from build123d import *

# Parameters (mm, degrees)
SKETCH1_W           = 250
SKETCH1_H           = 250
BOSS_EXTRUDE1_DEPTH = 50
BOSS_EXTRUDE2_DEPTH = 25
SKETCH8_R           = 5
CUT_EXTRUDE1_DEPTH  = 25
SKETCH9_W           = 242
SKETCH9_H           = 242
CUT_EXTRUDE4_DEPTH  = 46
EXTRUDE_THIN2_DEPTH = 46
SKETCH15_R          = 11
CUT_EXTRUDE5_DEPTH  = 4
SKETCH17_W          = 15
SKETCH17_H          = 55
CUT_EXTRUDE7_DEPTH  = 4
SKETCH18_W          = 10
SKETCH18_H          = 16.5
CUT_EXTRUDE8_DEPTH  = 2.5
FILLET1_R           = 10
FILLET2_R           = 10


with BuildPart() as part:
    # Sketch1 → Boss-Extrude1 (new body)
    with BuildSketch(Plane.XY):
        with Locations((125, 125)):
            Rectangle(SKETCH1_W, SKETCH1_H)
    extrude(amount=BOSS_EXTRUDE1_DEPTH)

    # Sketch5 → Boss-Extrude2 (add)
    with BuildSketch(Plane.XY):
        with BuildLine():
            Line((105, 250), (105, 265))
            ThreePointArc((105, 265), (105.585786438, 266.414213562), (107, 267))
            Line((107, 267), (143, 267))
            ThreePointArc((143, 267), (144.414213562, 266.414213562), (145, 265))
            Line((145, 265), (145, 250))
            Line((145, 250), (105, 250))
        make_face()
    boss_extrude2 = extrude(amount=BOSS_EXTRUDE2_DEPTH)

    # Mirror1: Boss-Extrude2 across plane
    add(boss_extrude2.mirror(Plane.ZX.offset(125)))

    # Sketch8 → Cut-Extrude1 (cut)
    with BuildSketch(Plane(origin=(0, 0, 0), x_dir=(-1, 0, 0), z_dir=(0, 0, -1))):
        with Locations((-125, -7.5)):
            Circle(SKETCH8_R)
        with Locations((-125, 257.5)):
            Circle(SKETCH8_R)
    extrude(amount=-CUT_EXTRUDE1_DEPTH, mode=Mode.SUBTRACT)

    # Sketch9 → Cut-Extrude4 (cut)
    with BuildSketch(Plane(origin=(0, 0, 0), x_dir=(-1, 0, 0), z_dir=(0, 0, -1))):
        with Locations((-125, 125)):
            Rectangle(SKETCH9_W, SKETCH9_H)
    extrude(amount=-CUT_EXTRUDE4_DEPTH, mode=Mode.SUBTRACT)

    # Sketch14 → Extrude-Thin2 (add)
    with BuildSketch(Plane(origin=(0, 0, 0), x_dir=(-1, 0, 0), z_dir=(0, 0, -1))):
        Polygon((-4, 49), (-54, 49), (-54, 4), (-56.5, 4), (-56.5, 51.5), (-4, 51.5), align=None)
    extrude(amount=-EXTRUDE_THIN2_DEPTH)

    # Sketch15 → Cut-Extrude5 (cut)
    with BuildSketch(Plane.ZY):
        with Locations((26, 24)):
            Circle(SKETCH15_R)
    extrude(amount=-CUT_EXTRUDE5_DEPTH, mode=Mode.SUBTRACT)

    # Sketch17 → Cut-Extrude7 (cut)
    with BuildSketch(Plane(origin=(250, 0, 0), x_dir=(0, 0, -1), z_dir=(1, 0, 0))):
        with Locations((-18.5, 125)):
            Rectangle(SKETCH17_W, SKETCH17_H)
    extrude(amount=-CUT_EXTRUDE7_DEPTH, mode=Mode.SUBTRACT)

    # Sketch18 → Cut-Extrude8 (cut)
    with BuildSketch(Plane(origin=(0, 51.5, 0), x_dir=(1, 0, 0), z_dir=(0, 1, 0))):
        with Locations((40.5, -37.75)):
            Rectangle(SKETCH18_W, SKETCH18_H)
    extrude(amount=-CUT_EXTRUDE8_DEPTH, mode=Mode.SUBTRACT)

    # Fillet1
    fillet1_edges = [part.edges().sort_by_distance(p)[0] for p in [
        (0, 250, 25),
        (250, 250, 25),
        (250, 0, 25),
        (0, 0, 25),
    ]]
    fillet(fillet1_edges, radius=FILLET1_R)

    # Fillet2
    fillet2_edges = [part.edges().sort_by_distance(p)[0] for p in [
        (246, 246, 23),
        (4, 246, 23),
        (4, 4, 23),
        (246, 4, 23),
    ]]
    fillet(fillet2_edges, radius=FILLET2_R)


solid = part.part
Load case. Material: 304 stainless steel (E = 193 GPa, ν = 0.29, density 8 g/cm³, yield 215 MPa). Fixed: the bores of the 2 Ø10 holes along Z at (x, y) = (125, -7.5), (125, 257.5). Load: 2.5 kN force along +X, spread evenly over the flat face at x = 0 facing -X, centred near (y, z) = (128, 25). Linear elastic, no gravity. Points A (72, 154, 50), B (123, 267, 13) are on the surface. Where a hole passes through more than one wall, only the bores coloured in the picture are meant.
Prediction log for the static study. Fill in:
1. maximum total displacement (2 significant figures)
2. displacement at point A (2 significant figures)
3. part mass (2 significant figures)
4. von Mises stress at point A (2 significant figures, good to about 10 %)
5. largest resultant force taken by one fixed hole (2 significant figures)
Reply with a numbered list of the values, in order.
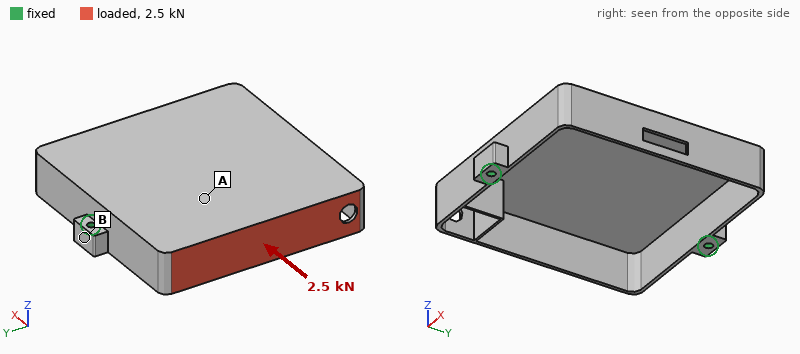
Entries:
1. 0.26 mm
2. 0.079 mm
3. 3.7 kg
4. 9.8 MPa
5. 1.3 kN
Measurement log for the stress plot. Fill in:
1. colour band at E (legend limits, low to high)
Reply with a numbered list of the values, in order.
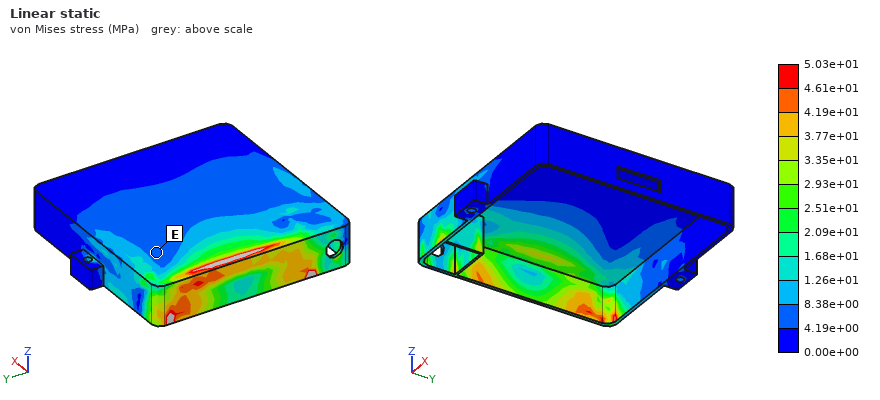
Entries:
1. 4.19e+00 to 8.38e+00 MPa
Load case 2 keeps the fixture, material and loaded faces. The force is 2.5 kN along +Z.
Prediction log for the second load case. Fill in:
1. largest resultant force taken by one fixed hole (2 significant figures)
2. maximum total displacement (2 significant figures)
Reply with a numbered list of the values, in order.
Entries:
1. 1.3 kN
2. 0.17 mm
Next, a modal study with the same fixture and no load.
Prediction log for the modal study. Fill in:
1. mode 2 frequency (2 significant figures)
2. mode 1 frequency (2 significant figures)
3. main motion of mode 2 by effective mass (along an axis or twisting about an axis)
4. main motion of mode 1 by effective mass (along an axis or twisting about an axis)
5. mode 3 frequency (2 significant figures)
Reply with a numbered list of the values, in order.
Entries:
1. 610 Hz
2. 460 Hz
3. along Y
4. along Z
5. 630 Hz
